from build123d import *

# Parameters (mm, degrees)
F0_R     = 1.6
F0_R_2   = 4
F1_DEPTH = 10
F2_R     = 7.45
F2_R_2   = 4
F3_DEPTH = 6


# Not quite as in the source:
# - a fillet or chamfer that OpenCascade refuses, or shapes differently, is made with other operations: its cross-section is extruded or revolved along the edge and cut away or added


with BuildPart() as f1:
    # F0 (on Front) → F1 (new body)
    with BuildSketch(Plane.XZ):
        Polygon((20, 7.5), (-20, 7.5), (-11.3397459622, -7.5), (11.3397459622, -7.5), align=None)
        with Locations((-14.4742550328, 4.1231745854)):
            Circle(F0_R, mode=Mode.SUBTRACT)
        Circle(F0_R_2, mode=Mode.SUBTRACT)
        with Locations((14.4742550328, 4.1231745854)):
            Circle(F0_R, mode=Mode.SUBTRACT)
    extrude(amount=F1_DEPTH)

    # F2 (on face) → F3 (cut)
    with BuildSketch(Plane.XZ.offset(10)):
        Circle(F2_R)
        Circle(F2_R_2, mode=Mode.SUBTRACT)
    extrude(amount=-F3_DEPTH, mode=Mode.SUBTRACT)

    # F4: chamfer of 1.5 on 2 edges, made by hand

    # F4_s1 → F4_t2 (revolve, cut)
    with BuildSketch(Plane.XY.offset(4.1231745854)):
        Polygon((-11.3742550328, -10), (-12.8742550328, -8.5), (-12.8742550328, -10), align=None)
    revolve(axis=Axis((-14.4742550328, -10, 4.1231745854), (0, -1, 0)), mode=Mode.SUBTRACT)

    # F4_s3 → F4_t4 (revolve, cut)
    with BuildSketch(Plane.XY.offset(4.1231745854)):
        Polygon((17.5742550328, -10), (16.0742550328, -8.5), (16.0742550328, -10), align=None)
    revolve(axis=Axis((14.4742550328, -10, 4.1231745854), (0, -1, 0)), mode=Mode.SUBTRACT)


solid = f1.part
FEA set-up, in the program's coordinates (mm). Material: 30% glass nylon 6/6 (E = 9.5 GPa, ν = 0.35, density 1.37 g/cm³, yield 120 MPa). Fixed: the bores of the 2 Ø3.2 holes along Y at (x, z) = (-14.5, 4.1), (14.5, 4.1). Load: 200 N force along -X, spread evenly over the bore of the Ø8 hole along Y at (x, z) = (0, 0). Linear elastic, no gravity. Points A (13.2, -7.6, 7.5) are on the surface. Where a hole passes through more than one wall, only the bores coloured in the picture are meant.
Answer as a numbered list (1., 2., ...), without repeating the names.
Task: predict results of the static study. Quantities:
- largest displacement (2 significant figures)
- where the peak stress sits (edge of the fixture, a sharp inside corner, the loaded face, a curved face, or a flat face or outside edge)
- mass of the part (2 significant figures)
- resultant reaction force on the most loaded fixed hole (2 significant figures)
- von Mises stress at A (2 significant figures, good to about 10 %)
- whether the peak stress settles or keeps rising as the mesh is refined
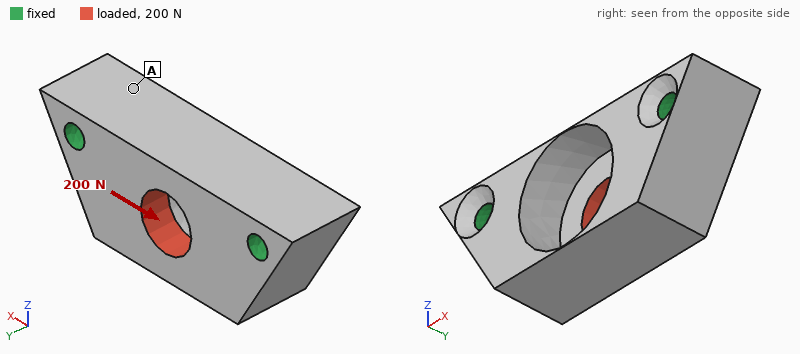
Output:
1. 5.2 µm
2. edge of the fixture
3. 4.5 g
4. 100 N
5. 0.61 MPa
6. keeps rising
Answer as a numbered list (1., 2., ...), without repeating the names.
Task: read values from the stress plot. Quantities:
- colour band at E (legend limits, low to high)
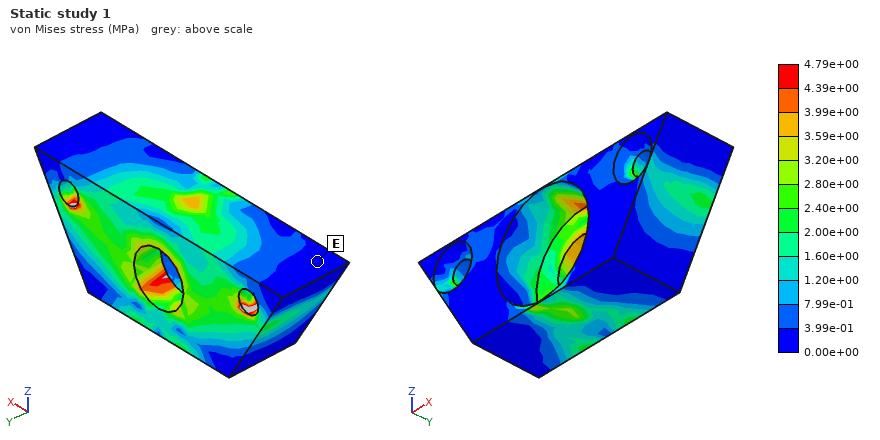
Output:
1. 0.00e+00 to 3.99e-01 MPa
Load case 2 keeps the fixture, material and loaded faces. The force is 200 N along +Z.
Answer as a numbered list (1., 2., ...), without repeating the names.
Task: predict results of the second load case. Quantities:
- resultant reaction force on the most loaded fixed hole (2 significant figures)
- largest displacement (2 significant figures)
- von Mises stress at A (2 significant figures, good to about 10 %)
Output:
1. 110 N
2. 12 µm
3. 2.0 MPa
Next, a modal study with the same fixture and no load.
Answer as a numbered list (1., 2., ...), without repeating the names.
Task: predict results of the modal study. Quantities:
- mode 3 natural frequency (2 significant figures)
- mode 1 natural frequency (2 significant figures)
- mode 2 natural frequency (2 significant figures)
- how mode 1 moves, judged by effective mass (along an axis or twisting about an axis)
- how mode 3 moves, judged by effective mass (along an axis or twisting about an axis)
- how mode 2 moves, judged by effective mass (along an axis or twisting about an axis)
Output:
1. 21 kHz
2. 15 kHz
3. 18 kHz
4. along Y
5. along Z
6. along X
